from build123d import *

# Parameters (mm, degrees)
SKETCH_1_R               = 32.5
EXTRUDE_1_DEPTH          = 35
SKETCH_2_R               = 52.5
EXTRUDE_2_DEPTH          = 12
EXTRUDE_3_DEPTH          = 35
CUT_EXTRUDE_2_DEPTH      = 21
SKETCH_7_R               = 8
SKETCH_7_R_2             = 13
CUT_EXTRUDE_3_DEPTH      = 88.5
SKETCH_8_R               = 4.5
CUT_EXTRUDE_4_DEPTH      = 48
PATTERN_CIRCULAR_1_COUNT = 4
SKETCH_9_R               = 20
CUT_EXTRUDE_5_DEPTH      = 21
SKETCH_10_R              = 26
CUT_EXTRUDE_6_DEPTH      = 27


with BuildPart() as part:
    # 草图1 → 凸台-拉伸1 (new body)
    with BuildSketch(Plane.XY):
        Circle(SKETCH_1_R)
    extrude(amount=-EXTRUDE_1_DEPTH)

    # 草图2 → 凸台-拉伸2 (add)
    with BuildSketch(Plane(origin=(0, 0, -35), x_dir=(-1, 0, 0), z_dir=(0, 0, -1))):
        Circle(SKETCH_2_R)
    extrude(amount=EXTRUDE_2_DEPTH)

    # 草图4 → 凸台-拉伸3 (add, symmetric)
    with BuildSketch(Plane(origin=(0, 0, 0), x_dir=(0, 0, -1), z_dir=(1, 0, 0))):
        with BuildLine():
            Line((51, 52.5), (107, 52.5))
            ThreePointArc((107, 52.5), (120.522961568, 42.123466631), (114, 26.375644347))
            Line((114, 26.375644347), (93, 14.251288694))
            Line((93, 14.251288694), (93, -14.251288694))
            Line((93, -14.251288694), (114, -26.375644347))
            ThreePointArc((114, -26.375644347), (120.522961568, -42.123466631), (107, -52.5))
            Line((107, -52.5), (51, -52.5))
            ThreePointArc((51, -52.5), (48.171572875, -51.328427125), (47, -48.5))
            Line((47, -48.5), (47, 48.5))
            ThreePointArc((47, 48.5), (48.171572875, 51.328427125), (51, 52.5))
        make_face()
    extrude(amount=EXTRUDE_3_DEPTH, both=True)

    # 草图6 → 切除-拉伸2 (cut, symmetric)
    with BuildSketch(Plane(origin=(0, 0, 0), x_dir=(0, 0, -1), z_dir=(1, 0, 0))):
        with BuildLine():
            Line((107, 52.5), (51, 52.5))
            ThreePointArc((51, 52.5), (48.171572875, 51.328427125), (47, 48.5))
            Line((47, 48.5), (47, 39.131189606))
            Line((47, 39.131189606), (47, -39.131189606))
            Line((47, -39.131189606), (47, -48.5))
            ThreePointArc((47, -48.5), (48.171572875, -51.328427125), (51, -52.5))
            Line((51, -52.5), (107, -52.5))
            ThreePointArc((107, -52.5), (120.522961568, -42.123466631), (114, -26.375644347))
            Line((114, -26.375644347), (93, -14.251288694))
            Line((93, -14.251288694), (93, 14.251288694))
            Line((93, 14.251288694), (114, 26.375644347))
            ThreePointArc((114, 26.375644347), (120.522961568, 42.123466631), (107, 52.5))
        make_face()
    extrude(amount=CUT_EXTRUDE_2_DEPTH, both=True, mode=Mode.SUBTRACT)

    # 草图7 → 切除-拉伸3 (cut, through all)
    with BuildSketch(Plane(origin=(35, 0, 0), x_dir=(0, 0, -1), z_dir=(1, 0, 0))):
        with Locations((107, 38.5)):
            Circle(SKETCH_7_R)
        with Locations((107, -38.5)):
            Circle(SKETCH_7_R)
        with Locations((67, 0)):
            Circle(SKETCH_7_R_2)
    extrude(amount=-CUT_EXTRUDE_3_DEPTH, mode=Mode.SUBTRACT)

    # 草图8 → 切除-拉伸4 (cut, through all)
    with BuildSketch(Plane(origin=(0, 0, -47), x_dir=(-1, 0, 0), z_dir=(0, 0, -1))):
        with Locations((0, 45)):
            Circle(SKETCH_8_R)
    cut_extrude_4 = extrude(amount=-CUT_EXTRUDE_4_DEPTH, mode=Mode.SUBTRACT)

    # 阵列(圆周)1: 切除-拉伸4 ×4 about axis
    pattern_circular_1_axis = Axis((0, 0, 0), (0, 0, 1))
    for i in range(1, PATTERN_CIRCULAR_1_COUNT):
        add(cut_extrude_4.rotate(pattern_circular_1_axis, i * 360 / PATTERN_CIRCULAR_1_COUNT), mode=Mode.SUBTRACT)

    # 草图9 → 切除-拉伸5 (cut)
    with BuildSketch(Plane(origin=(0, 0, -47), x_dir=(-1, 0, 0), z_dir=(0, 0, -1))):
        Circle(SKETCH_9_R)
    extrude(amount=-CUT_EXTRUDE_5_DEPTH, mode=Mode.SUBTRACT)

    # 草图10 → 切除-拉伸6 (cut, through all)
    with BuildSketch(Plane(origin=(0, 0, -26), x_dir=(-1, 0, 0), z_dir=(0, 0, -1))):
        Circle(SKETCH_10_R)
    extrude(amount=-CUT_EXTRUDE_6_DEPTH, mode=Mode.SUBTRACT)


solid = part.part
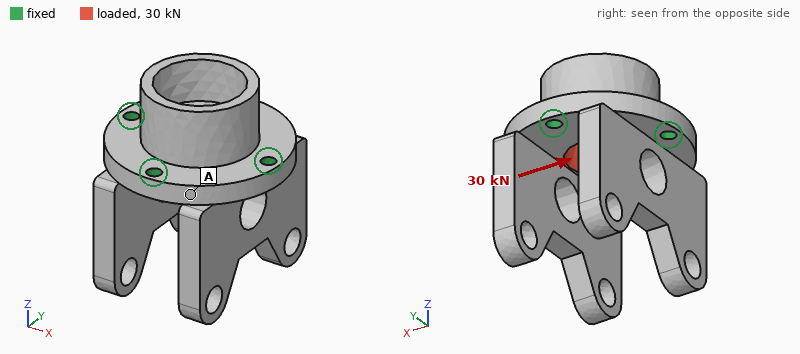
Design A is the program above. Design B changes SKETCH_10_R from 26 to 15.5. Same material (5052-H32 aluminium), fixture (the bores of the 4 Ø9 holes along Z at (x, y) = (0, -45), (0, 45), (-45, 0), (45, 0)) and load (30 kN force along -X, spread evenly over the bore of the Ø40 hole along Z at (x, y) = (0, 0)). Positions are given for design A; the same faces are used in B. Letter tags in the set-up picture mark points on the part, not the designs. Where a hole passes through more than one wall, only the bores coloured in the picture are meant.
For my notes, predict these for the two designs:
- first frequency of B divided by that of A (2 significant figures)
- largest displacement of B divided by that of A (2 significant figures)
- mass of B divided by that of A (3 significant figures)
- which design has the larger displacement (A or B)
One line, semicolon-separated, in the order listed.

1.0; 0.90; 1.12; A
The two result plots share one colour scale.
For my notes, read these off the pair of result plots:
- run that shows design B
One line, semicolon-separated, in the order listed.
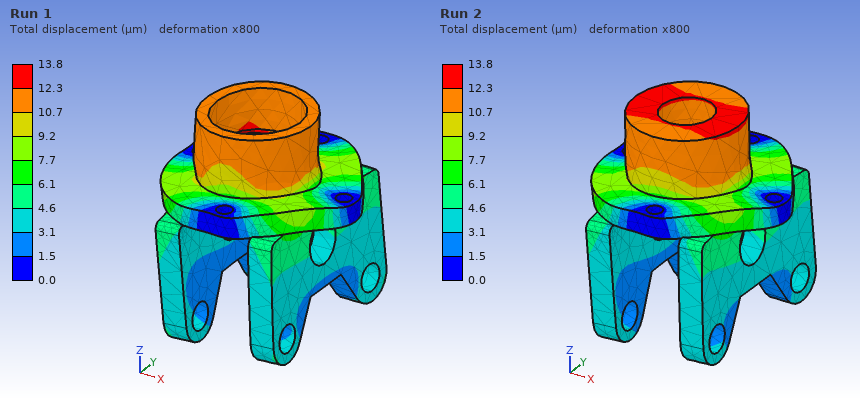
Run 2
